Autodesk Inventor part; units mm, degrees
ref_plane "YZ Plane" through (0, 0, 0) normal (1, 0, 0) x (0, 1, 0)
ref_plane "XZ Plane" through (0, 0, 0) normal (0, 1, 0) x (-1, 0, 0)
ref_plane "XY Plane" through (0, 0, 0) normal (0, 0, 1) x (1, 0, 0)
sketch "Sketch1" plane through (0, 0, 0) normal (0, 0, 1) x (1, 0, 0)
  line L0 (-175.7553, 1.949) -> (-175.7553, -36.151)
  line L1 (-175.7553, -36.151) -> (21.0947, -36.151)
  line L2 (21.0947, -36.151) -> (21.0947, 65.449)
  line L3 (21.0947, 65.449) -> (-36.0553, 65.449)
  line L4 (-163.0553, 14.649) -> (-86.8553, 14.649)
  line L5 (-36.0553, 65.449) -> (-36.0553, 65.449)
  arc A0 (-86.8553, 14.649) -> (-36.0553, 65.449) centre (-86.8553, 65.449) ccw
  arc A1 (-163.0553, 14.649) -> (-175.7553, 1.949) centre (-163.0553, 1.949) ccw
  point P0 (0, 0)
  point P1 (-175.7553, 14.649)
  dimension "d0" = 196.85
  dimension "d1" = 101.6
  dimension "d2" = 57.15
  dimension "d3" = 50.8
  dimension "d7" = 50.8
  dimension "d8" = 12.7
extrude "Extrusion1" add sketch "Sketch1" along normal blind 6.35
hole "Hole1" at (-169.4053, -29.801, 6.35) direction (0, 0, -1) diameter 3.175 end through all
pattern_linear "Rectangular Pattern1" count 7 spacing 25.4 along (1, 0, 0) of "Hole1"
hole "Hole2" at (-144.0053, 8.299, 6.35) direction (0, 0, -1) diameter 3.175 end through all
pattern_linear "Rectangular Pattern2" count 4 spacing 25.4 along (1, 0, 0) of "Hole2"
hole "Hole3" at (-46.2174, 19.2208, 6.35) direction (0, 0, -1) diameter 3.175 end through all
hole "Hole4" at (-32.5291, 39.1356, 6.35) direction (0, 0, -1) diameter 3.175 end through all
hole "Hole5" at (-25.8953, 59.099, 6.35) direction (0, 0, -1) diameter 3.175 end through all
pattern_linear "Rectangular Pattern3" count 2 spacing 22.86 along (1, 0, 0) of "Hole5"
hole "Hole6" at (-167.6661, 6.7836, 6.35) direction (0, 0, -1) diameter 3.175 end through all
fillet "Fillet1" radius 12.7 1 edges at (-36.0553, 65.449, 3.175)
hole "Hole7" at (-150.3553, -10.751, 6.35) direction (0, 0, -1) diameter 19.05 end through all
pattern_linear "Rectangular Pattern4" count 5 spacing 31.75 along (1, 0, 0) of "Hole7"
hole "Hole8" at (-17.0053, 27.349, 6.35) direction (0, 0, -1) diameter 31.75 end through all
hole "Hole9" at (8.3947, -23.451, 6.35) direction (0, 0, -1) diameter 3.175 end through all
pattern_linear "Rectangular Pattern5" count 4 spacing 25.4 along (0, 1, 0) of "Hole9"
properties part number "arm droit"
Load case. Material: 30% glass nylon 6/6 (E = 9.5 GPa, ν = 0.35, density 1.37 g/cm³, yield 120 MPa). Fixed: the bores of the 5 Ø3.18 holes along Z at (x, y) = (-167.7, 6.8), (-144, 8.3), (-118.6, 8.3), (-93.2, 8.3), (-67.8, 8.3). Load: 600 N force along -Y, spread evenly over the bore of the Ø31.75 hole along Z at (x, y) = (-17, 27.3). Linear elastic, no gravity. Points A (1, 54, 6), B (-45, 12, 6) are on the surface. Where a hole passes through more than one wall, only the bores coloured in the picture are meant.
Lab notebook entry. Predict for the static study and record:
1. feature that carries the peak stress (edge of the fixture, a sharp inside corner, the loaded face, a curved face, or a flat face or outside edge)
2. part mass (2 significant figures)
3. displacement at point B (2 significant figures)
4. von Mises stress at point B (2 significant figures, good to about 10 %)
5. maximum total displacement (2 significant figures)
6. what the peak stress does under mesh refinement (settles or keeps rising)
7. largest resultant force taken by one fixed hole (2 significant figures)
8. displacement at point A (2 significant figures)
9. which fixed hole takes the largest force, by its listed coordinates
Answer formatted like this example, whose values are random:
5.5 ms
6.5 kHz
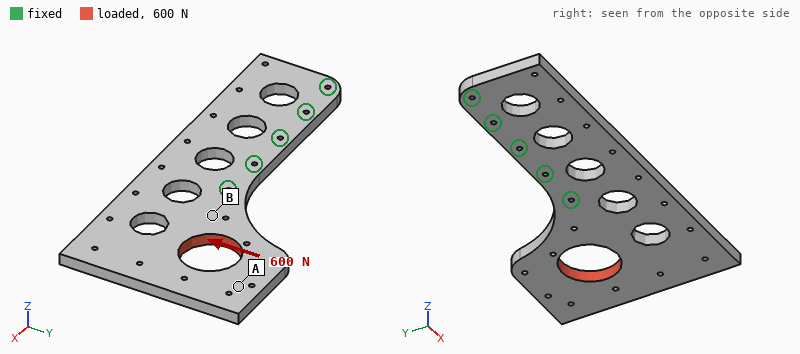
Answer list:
edge of the fixture
96 g
0.090 mm
4.3 MPa
0.36 mm
keeps rising
1.1 kN
0.29 mm
(-67.8, 8.3)
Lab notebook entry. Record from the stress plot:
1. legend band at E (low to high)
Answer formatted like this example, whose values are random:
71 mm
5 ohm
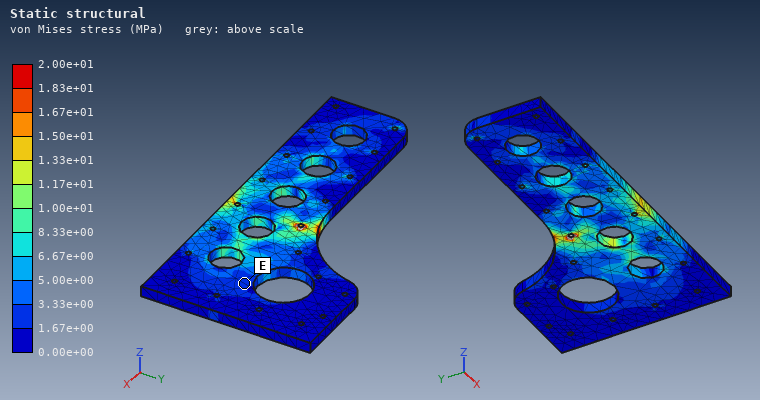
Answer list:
1.67e+00 to 3.33e+00 MPa
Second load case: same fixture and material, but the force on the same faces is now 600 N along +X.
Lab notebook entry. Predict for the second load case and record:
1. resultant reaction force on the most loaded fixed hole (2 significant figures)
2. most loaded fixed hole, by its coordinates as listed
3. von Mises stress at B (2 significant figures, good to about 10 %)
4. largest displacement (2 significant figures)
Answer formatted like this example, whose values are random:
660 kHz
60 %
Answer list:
700 N
(-67.8, 8.3)
3.9 MPa
0.19 mm
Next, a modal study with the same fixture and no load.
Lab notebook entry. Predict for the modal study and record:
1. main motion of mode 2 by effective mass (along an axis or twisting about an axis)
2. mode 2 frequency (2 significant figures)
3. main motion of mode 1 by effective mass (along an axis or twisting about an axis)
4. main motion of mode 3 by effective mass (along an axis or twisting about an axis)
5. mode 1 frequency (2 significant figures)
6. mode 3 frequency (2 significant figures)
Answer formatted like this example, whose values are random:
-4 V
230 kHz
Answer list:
twisting about X
370 Hz
along Z
along Y
210 Hz
1000 Hz
